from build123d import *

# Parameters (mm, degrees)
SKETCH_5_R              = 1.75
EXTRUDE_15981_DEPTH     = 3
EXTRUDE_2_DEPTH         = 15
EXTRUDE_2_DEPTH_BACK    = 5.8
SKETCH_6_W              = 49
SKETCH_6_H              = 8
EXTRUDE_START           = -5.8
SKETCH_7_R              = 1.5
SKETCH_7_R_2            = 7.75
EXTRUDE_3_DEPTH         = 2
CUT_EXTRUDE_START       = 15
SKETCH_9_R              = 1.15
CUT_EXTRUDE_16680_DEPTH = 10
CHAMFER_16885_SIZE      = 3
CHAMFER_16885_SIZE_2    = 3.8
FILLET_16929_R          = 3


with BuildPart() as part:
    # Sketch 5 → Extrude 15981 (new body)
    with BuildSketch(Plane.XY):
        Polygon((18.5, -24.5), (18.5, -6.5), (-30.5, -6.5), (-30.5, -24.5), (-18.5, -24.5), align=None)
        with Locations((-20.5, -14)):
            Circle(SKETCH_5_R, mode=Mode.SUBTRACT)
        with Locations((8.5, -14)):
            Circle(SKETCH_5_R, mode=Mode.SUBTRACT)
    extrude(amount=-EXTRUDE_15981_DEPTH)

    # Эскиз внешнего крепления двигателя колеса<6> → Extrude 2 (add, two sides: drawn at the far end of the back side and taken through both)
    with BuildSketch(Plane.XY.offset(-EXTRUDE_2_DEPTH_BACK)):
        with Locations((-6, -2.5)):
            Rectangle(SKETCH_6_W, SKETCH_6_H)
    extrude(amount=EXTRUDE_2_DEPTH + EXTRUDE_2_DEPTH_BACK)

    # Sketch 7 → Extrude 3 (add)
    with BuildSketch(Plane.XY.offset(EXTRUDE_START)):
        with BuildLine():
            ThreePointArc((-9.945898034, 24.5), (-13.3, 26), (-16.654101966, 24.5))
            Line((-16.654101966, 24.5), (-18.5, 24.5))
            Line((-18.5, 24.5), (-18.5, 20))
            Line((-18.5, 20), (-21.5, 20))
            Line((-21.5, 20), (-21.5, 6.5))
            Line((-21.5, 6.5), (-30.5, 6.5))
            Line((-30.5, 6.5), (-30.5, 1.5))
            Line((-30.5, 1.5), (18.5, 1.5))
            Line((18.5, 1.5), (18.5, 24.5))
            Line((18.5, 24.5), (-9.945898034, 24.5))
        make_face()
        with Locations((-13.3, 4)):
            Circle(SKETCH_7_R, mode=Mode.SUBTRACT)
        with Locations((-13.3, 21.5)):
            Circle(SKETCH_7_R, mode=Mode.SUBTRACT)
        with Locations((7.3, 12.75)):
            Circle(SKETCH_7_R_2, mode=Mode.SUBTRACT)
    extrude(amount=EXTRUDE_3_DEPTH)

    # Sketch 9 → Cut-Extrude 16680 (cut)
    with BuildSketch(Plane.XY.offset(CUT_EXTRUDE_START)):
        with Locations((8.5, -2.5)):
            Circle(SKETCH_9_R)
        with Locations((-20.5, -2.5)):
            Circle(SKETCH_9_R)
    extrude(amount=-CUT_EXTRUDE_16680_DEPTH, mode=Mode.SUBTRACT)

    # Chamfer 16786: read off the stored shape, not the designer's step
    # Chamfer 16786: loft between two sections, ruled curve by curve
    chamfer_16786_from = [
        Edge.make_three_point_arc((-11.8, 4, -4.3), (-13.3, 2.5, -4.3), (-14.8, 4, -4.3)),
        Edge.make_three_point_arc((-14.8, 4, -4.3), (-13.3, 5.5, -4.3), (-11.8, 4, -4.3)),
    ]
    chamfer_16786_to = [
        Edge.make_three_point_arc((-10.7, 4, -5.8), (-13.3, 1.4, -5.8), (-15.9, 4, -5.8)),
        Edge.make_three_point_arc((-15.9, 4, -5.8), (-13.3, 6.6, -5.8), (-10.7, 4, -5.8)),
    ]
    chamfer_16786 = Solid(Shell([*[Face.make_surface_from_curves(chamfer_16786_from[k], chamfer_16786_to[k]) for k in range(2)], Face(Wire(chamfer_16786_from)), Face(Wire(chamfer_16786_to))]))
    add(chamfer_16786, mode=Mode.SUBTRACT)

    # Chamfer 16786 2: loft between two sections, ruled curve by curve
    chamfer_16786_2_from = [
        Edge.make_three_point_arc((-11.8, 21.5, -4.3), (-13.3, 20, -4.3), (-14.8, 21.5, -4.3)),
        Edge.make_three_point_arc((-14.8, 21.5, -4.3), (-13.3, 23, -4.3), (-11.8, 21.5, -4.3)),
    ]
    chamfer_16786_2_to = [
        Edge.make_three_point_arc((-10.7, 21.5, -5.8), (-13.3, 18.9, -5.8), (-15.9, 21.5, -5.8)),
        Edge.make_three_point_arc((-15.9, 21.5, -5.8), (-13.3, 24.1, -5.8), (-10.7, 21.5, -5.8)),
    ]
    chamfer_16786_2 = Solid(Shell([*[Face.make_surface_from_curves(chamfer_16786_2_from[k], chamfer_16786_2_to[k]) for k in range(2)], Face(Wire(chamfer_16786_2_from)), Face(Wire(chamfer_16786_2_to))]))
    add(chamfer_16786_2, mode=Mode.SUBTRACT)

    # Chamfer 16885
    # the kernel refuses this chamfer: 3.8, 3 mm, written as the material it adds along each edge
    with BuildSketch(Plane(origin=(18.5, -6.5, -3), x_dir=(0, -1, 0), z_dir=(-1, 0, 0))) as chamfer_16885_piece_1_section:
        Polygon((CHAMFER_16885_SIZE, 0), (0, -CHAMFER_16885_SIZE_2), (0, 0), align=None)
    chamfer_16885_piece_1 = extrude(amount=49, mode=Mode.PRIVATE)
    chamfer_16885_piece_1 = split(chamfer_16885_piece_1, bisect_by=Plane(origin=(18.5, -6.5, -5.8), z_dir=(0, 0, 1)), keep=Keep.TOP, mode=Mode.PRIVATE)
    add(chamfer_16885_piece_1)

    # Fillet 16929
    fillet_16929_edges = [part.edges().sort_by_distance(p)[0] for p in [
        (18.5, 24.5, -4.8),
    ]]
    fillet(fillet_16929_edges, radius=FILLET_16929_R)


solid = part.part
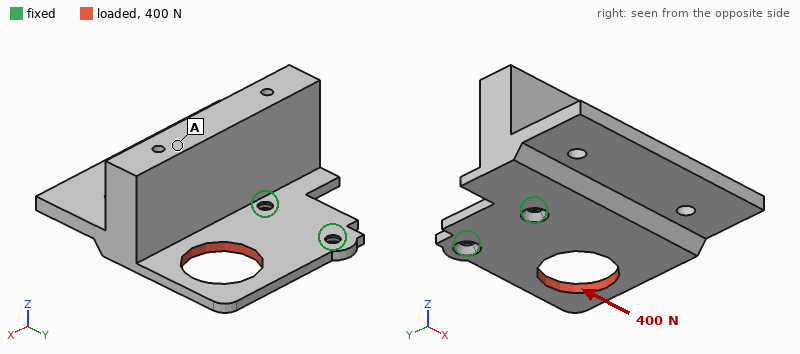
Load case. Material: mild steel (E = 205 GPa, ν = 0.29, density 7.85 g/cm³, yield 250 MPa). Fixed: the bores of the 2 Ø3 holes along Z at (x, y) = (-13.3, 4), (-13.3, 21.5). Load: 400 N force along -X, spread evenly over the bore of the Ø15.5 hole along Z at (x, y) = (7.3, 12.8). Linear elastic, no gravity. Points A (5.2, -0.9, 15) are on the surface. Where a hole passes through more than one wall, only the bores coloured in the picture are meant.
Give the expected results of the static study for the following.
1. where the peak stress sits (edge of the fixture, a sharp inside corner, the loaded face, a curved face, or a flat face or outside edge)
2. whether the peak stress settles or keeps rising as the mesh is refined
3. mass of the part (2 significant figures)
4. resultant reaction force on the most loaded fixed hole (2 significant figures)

edge of the fixture
keeps rising
97 g
200 N
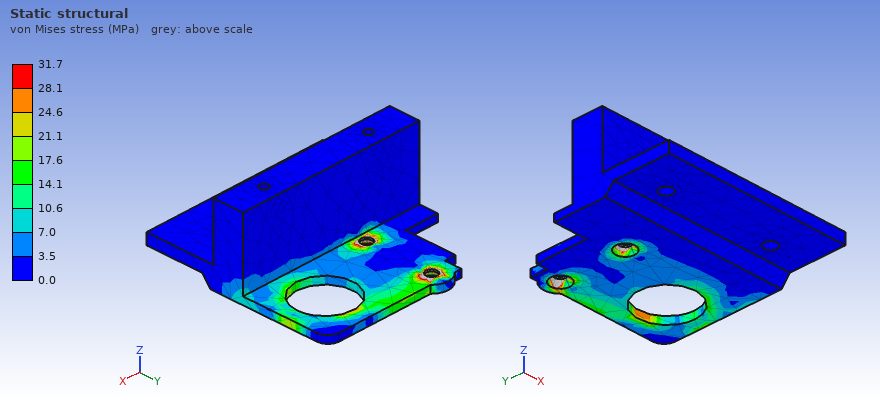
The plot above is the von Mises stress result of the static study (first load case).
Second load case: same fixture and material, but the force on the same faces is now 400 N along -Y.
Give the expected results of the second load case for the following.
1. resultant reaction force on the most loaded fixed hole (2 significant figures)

490 N
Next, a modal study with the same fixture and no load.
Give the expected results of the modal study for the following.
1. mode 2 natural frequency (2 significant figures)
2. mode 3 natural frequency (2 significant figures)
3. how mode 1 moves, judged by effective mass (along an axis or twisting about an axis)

980 Hz
4000 Hz
along Z
